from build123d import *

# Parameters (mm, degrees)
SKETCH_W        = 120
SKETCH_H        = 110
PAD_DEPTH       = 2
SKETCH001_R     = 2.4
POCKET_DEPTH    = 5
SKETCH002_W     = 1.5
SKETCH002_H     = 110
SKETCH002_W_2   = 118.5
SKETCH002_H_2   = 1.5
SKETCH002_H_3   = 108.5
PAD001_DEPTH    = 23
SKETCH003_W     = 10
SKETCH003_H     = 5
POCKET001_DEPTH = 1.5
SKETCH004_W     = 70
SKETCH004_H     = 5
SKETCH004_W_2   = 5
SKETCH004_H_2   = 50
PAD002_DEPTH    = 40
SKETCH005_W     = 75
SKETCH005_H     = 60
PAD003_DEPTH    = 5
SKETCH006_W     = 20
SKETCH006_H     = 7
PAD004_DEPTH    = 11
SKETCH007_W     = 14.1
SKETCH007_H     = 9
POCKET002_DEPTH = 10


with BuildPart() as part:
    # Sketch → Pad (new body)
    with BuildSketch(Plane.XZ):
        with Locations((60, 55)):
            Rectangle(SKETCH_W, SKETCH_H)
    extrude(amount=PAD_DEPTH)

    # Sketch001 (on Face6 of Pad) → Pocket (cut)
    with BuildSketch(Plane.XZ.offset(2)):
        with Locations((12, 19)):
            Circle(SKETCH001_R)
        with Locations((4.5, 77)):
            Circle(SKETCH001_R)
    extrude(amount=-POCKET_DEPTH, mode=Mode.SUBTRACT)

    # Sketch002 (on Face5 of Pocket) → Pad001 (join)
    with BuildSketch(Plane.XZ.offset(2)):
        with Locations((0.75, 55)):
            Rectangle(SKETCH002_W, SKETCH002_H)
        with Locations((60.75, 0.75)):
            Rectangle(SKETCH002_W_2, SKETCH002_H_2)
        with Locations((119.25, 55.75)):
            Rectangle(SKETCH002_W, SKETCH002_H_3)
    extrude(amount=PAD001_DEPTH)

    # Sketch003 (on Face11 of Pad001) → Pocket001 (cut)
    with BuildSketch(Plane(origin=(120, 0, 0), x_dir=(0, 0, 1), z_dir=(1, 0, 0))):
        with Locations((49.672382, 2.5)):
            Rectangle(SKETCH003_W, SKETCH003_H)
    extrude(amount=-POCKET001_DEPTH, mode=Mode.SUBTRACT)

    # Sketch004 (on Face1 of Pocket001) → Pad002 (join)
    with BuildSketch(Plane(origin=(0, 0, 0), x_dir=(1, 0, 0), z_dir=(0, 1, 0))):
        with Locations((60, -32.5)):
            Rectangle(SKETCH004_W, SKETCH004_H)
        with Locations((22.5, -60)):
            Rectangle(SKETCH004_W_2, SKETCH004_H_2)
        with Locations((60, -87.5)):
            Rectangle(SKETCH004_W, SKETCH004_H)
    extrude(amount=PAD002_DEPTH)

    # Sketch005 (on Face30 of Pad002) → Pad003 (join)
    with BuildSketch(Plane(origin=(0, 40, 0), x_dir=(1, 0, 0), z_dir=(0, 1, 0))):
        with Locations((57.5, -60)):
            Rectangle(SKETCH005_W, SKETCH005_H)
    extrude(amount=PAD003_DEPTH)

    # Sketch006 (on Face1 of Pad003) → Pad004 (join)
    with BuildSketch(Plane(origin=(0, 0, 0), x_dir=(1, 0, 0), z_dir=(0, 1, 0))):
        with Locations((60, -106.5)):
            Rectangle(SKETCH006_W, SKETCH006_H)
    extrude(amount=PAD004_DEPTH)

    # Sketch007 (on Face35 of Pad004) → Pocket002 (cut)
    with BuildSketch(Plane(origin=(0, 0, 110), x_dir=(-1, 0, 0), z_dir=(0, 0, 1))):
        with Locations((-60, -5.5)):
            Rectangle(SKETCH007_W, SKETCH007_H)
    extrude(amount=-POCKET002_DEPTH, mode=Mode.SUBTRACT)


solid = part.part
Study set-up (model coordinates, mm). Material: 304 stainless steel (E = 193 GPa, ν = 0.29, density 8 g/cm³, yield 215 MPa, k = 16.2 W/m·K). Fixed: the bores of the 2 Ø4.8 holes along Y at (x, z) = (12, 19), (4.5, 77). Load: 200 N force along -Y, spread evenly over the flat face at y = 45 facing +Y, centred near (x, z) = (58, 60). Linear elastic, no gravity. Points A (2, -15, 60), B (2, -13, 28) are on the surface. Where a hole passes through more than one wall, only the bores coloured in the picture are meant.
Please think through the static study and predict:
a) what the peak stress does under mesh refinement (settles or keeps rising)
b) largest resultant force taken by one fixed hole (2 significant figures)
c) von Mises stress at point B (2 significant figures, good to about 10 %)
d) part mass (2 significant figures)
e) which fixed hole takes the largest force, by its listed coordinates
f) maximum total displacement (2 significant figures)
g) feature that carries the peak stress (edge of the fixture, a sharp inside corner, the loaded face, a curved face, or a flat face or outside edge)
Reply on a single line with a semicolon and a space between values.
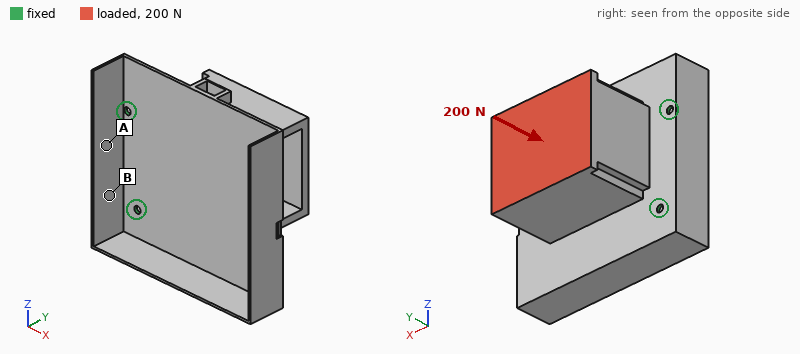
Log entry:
keeps rising; 130 N; 22 MPa; 790 g; (4.5, 77); 0.88 mm; edge of the fixture
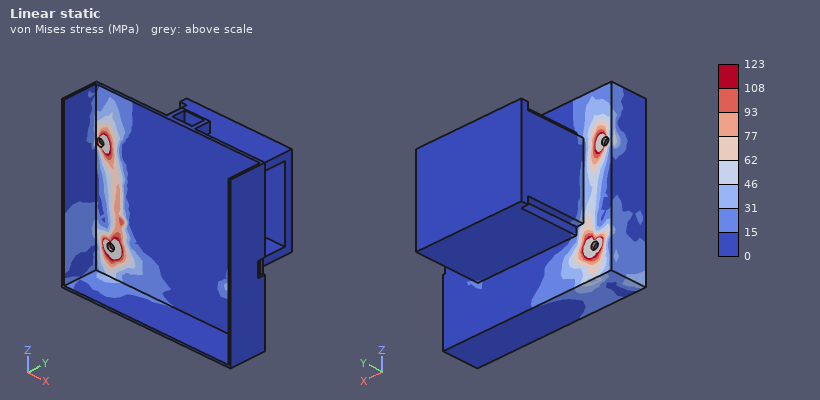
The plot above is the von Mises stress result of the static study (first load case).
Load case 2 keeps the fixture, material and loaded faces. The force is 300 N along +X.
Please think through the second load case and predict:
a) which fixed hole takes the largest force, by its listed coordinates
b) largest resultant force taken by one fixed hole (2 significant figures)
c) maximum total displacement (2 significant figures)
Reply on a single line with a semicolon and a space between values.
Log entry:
(4.5, 77); 230 N; 1.3 mm
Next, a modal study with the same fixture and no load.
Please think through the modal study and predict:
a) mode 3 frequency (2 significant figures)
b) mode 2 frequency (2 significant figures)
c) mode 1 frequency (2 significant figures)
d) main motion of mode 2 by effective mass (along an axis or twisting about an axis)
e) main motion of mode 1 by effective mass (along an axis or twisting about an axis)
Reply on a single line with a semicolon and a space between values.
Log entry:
960 Hz; 520 Hz; 110 Hz; along Z; along Y
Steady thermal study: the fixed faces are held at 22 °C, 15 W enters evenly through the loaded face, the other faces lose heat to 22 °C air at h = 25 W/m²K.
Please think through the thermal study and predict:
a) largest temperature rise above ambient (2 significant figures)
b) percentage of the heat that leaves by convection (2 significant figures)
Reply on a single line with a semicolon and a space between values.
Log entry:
39 K; 96 %
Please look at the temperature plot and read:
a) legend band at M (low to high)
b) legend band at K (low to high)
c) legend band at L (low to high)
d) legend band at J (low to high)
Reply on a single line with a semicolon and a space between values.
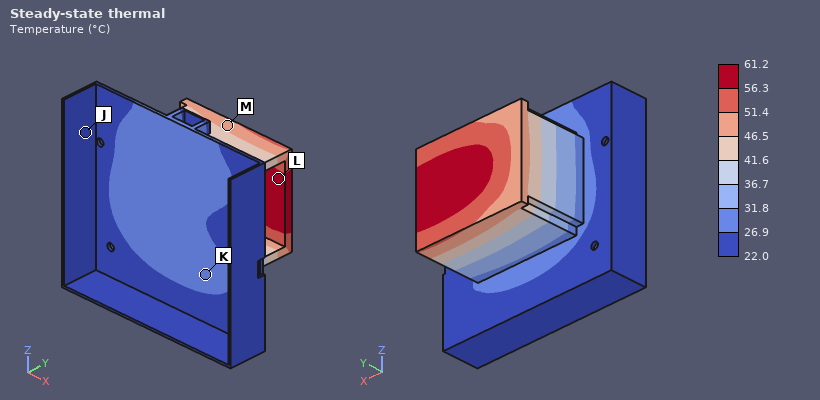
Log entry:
46.5 to 51.4 °C; 26.9 to 31.8 °C; 56.3 to 61.2 °C; 22.0 to 26.9 °C
